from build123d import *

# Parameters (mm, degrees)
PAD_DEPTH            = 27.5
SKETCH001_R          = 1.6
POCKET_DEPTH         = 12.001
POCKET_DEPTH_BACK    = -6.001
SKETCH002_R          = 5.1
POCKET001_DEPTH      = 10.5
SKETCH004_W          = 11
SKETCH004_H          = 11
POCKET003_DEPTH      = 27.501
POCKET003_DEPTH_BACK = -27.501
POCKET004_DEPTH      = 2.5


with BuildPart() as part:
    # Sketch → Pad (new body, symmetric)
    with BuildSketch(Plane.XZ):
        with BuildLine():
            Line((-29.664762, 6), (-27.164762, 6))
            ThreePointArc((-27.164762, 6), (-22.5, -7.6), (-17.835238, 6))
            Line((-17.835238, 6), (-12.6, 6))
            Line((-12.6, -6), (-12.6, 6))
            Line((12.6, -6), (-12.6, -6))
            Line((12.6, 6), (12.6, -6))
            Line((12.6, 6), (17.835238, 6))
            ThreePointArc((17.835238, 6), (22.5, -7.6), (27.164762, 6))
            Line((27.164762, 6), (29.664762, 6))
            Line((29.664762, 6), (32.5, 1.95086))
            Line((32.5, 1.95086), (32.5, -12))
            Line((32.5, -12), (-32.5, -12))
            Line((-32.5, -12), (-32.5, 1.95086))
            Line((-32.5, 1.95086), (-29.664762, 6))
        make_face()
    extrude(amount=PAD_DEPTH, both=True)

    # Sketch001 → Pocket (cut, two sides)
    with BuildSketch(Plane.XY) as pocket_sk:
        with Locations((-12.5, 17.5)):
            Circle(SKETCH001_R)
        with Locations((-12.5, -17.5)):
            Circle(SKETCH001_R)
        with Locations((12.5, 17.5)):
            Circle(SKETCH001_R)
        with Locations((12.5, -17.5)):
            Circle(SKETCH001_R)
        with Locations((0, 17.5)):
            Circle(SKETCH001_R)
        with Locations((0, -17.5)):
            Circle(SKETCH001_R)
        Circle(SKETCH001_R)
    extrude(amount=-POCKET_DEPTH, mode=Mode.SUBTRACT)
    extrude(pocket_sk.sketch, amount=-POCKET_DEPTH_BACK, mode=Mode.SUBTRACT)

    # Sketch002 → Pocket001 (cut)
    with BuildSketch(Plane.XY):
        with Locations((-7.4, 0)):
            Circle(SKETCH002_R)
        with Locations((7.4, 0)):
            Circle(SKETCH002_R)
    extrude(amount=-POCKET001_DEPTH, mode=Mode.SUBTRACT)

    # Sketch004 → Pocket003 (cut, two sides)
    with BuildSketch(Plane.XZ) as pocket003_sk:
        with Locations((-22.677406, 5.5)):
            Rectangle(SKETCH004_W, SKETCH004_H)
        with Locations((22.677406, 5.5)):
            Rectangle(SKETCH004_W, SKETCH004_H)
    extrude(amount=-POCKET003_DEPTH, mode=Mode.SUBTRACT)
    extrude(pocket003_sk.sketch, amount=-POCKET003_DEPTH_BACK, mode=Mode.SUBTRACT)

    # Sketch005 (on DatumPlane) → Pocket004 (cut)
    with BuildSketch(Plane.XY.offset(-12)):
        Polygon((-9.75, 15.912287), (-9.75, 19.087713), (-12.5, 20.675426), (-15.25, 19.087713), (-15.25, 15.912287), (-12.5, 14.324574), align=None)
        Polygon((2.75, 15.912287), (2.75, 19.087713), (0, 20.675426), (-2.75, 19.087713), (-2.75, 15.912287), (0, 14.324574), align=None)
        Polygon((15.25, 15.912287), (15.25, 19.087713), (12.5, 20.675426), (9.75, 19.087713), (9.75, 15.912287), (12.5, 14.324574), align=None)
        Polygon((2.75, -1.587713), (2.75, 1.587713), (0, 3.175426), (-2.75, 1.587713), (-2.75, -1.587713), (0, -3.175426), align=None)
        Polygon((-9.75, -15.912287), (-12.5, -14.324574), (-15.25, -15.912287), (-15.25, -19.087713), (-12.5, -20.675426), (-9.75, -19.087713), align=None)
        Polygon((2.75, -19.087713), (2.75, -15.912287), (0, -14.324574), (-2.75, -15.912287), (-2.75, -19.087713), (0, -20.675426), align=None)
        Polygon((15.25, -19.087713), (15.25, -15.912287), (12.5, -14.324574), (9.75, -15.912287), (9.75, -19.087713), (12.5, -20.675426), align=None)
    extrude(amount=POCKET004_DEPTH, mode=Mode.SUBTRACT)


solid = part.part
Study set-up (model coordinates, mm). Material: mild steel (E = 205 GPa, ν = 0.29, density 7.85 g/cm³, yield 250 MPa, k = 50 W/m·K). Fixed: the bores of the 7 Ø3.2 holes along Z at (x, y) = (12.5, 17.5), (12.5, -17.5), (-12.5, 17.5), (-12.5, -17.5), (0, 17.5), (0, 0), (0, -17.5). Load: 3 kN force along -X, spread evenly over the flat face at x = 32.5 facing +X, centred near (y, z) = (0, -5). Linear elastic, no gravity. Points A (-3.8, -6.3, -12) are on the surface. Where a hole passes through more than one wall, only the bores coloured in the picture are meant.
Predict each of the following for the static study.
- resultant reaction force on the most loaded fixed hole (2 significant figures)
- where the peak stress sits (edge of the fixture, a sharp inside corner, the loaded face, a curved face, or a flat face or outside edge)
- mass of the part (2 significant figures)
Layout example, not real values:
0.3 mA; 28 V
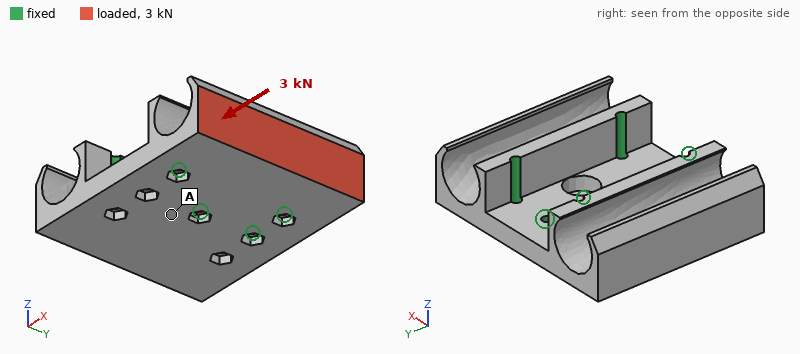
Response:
1.2 kN; a curved face; 210 g
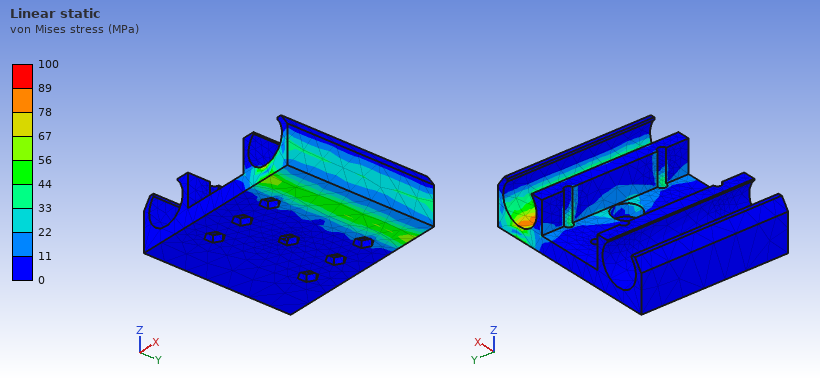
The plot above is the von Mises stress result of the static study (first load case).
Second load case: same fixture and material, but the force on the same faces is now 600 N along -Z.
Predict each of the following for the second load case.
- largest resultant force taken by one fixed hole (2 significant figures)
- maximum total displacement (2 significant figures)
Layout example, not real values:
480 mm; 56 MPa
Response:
570 N; 17 µm
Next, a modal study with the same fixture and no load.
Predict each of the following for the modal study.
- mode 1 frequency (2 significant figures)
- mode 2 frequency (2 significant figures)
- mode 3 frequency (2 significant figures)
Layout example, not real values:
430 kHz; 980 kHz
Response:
6600 Hz; 6600 Hz; 9200 Hz
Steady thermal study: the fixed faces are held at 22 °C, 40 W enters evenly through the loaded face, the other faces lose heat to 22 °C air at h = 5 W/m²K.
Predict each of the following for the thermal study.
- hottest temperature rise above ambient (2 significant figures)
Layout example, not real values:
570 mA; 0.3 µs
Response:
70 K
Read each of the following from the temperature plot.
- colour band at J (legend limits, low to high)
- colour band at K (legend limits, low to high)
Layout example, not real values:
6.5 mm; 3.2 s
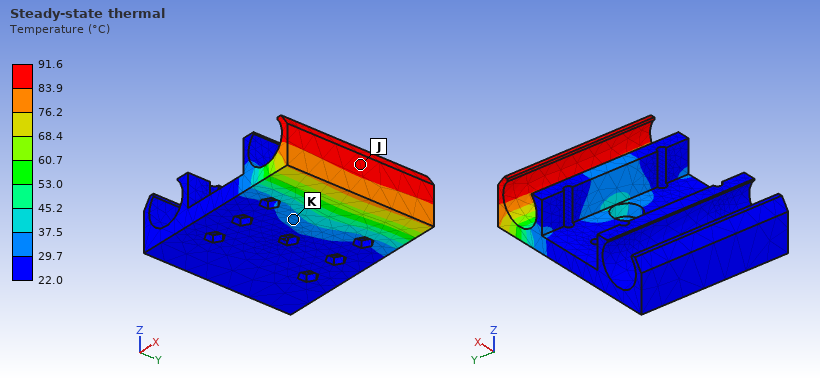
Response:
83.9 to 91.6 °C; 29.7 to 37.5 °C
